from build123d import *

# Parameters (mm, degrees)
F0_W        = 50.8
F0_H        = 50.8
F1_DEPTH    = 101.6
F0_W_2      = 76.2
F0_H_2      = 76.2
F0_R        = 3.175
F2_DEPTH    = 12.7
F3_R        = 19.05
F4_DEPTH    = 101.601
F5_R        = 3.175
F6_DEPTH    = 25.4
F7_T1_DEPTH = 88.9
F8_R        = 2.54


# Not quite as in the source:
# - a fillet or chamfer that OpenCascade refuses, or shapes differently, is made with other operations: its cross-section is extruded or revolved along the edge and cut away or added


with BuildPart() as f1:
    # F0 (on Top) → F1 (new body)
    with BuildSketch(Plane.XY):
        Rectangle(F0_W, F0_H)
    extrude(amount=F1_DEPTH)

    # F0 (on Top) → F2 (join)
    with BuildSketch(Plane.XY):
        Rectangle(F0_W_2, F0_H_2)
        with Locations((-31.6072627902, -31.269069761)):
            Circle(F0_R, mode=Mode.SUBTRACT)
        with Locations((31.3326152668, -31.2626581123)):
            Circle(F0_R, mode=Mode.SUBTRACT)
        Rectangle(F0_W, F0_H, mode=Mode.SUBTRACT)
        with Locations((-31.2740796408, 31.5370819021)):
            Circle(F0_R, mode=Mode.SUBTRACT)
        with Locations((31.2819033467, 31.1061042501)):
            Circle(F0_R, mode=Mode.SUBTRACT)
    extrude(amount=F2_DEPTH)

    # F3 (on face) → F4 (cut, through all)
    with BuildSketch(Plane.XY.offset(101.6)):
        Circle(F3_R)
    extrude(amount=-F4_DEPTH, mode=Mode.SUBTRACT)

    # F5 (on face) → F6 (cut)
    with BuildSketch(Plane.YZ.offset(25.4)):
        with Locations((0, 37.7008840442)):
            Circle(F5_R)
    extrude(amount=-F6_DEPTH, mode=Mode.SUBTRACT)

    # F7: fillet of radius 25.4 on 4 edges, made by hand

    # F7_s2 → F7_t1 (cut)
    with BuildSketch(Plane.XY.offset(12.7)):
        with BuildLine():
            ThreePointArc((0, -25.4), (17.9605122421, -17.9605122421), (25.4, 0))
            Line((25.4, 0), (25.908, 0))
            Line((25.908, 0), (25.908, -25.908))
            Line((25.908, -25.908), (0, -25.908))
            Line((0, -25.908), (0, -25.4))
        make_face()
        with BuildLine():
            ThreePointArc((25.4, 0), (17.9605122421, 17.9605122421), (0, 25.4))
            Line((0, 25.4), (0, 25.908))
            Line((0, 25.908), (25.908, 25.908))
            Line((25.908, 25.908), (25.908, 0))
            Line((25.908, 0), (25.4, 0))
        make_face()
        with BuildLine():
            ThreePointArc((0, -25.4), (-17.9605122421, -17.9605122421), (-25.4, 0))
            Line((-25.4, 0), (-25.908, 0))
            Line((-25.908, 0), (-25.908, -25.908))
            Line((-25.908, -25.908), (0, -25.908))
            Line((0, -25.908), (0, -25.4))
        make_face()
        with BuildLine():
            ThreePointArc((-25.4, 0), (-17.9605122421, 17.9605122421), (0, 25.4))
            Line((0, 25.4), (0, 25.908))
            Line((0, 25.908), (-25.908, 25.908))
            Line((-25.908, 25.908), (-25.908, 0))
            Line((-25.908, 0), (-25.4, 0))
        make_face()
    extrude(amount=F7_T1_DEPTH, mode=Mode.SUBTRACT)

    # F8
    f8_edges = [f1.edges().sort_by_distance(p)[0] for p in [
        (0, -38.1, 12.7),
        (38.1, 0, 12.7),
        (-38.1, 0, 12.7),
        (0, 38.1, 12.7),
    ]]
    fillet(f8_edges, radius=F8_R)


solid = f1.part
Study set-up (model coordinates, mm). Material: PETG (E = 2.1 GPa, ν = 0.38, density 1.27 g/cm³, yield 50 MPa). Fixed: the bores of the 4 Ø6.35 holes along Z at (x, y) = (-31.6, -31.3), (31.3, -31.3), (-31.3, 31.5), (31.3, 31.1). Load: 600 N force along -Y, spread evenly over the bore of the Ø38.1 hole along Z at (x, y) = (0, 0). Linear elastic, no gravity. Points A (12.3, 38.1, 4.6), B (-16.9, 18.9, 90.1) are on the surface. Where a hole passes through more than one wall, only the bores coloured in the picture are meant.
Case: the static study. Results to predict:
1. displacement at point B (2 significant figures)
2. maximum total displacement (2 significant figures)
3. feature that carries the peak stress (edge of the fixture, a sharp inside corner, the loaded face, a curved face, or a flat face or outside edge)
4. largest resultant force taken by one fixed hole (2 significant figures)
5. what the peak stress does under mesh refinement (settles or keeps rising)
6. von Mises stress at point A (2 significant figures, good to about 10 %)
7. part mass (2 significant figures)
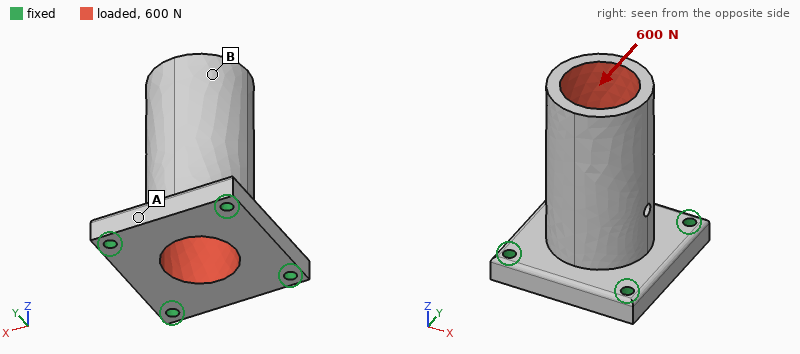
0.37 mm
0.43 mm
edge of the fixture
300 N
keeps rising
1.6 MPa
170 g
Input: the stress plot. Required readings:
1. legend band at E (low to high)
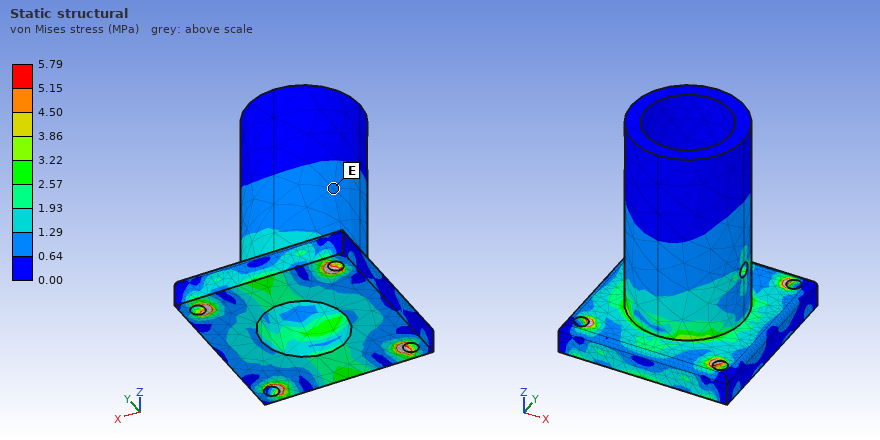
0.64 to 1.29 MPa
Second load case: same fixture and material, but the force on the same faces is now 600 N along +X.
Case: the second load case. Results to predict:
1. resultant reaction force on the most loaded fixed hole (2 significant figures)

300 N
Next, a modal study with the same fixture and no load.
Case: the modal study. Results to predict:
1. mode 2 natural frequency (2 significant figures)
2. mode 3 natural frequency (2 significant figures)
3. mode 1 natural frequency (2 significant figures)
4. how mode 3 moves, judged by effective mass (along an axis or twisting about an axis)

660 Hz
1600 Hz
660 Hz
along Z
